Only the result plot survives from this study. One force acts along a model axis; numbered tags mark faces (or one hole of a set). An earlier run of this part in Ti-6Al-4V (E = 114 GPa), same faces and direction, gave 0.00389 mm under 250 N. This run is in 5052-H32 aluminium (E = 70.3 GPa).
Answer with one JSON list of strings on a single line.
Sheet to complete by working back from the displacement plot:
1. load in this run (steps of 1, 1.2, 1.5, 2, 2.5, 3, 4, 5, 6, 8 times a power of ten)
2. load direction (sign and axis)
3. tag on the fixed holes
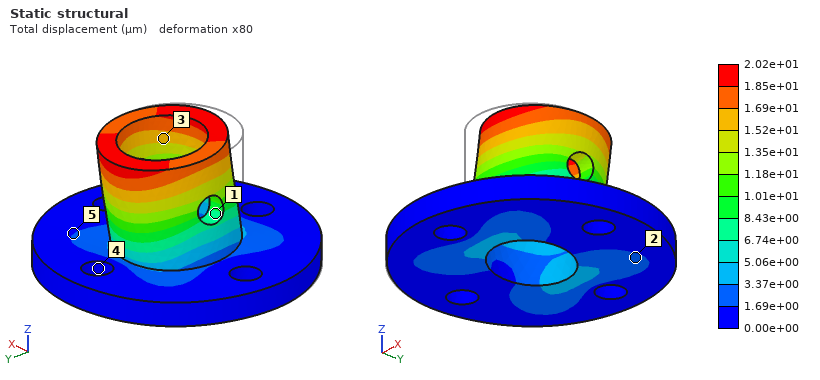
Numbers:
["800 N", "+Y", "4"]
